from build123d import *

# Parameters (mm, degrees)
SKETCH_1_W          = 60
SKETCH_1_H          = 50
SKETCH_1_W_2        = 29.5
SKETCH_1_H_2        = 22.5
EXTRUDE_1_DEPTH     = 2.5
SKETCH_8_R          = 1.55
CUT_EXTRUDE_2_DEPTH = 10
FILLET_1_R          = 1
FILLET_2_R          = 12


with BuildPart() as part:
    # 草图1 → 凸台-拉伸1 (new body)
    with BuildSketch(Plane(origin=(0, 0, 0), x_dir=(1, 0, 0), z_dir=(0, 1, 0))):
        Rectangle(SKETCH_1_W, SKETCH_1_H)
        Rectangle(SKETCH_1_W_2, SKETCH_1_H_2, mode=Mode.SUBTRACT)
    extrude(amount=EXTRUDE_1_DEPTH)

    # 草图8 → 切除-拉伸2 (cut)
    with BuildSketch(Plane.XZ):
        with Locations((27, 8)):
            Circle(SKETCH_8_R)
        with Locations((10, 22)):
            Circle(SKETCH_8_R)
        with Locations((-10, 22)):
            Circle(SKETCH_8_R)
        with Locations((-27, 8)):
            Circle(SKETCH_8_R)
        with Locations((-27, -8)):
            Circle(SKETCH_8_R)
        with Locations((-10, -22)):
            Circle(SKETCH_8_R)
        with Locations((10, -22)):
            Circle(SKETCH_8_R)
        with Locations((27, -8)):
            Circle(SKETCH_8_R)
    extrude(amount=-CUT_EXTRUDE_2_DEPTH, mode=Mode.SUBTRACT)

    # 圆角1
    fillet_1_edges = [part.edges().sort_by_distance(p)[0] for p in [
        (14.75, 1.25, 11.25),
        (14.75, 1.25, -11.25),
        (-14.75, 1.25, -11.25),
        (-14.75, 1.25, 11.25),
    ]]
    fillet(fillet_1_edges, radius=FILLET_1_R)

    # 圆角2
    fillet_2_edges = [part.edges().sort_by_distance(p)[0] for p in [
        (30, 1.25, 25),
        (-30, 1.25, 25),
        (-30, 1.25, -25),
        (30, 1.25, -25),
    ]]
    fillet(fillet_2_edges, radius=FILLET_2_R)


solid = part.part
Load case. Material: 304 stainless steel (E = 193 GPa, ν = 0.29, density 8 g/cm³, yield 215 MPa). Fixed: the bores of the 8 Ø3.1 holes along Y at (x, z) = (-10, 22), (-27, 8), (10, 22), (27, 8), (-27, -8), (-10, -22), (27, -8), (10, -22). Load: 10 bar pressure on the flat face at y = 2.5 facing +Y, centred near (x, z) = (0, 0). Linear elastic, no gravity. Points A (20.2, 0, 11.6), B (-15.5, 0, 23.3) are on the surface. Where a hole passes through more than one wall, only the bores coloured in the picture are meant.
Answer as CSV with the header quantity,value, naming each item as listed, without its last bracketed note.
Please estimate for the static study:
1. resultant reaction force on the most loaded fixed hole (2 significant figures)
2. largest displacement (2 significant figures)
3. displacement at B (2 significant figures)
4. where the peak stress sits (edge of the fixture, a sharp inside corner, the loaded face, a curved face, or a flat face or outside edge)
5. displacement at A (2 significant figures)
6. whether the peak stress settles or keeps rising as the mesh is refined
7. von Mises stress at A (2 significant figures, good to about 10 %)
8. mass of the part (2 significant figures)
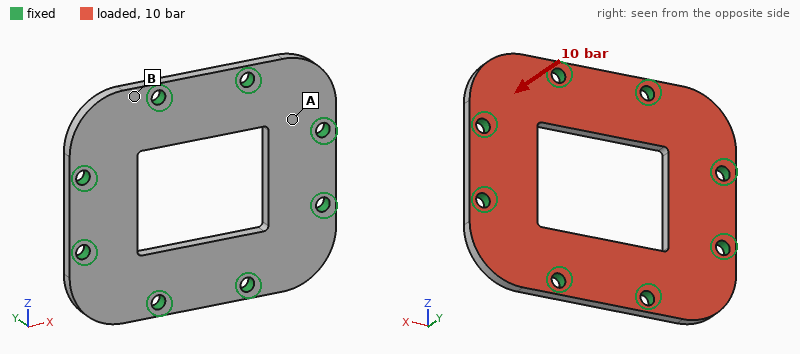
quantity,value
resultant reaction force on the most loaded fixed hole,280 N
largest displacement,8.3 µm
displacement at B,1.6 µm
where the peak stress sits,edge of the fixture
displacement at A,3.1 µm
whether the peak stress settles or keeps rising as the mesh is refined,keeps rising
von Mises stress at A,26 MPa
mass of the part,43 g
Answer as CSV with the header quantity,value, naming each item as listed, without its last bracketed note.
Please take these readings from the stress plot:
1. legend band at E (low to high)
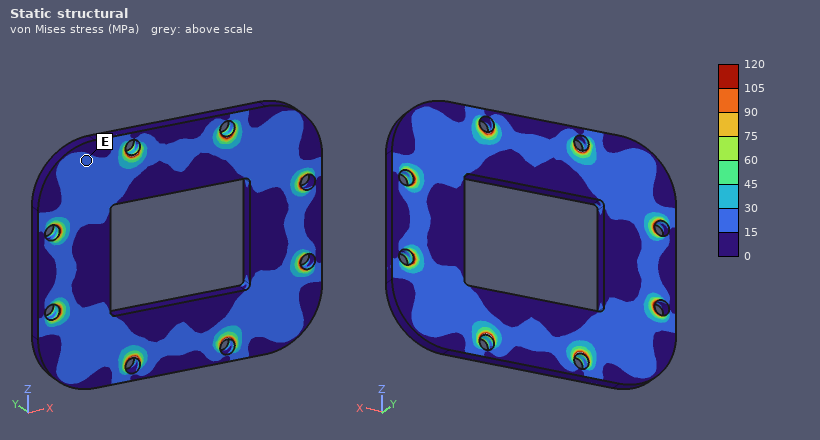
quantity,value
legend band at E,15 to 30 MPa
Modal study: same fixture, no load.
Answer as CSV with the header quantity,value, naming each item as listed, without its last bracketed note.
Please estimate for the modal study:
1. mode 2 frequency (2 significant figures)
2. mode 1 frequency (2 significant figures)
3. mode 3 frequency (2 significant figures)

quantity,value
mode 2 frequency,16 kHz
mode 1 frequency,15 kHz
mode 3 frequency,16 kHz
